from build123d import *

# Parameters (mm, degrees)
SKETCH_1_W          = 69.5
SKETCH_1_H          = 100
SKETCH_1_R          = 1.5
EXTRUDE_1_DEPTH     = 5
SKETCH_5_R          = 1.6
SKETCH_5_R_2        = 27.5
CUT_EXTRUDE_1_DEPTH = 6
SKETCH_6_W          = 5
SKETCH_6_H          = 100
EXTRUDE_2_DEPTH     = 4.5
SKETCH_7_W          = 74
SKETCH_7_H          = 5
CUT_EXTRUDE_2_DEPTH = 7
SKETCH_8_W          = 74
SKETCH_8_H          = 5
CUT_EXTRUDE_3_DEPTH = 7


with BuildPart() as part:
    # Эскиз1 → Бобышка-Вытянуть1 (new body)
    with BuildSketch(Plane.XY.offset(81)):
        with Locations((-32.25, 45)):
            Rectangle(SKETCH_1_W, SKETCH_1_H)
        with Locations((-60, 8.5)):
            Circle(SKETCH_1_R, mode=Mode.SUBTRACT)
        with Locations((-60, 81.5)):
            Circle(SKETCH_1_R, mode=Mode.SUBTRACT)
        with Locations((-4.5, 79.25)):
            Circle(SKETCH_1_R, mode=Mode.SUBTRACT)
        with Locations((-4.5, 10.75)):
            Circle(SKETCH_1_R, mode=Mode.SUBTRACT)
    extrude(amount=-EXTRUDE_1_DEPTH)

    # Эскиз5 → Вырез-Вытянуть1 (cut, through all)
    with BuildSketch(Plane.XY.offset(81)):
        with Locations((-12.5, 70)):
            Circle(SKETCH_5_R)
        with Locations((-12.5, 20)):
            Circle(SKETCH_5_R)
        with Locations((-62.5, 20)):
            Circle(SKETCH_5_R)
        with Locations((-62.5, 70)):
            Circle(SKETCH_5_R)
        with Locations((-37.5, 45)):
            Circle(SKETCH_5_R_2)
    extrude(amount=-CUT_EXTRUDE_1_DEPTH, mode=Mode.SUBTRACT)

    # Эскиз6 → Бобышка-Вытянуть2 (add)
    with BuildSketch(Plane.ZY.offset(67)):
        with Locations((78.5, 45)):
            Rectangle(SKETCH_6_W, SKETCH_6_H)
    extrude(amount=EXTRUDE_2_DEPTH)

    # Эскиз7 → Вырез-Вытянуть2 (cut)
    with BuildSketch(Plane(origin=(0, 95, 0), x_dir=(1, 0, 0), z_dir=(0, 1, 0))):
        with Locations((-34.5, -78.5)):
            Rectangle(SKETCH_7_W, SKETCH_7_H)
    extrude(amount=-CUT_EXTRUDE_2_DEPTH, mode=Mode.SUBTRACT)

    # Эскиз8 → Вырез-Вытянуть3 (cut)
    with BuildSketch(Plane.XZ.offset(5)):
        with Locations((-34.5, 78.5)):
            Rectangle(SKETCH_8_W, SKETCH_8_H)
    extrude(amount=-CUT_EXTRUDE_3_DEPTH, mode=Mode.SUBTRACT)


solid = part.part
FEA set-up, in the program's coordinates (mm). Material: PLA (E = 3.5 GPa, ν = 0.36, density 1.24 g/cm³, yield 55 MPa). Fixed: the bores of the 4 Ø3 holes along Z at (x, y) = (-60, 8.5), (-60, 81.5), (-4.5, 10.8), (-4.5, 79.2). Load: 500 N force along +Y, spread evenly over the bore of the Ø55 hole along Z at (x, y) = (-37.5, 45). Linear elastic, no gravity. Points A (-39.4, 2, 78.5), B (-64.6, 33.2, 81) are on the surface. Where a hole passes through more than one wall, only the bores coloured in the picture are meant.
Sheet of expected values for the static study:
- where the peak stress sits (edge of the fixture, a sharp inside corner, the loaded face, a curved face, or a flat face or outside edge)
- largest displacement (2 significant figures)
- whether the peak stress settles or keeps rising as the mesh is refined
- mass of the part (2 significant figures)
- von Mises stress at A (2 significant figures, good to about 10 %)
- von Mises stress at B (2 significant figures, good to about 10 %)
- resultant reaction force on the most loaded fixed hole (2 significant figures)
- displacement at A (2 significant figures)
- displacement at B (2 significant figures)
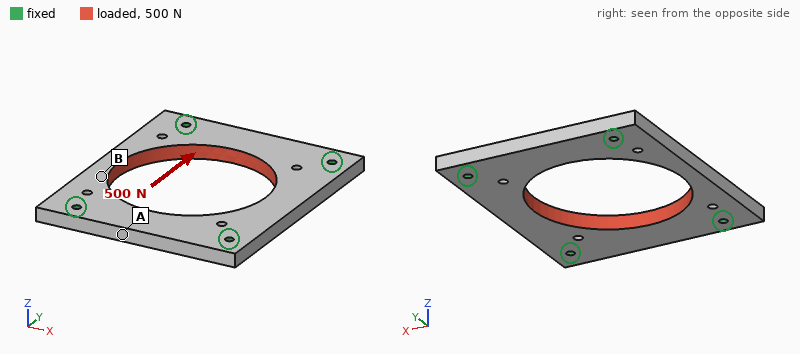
edge of the fixture
25 µm
keeps rising
24 g
1.8 MPa
0.86 MPa
140 N
22 µm
9.9 µm
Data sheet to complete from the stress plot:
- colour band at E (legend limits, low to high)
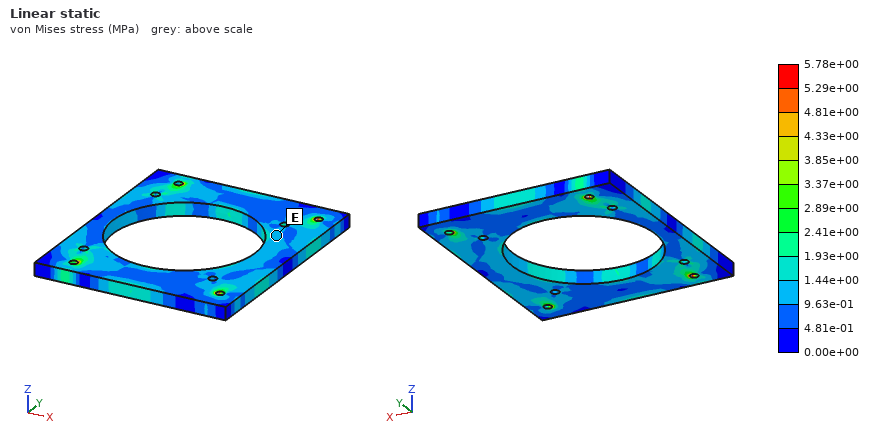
9.63e-01 to 1.44e+00 MPa
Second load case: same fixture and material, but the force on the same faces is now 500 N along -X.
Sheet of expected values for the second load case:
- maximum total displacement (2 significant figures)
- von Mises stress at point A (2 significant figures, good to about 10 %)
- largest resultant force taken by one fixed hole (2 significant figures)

70 µm
1.3 MPa
130 N
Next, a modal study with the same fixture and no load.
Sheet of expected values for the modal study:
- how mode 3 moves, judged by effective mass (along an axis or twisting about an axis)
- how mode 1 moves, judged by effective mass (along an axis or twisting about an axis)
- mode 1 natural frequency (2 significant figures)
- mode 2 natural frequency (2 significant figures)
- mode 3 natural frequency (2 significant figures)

along Z
along Z
1800 Hz
1800 Hz
2500 Hz
